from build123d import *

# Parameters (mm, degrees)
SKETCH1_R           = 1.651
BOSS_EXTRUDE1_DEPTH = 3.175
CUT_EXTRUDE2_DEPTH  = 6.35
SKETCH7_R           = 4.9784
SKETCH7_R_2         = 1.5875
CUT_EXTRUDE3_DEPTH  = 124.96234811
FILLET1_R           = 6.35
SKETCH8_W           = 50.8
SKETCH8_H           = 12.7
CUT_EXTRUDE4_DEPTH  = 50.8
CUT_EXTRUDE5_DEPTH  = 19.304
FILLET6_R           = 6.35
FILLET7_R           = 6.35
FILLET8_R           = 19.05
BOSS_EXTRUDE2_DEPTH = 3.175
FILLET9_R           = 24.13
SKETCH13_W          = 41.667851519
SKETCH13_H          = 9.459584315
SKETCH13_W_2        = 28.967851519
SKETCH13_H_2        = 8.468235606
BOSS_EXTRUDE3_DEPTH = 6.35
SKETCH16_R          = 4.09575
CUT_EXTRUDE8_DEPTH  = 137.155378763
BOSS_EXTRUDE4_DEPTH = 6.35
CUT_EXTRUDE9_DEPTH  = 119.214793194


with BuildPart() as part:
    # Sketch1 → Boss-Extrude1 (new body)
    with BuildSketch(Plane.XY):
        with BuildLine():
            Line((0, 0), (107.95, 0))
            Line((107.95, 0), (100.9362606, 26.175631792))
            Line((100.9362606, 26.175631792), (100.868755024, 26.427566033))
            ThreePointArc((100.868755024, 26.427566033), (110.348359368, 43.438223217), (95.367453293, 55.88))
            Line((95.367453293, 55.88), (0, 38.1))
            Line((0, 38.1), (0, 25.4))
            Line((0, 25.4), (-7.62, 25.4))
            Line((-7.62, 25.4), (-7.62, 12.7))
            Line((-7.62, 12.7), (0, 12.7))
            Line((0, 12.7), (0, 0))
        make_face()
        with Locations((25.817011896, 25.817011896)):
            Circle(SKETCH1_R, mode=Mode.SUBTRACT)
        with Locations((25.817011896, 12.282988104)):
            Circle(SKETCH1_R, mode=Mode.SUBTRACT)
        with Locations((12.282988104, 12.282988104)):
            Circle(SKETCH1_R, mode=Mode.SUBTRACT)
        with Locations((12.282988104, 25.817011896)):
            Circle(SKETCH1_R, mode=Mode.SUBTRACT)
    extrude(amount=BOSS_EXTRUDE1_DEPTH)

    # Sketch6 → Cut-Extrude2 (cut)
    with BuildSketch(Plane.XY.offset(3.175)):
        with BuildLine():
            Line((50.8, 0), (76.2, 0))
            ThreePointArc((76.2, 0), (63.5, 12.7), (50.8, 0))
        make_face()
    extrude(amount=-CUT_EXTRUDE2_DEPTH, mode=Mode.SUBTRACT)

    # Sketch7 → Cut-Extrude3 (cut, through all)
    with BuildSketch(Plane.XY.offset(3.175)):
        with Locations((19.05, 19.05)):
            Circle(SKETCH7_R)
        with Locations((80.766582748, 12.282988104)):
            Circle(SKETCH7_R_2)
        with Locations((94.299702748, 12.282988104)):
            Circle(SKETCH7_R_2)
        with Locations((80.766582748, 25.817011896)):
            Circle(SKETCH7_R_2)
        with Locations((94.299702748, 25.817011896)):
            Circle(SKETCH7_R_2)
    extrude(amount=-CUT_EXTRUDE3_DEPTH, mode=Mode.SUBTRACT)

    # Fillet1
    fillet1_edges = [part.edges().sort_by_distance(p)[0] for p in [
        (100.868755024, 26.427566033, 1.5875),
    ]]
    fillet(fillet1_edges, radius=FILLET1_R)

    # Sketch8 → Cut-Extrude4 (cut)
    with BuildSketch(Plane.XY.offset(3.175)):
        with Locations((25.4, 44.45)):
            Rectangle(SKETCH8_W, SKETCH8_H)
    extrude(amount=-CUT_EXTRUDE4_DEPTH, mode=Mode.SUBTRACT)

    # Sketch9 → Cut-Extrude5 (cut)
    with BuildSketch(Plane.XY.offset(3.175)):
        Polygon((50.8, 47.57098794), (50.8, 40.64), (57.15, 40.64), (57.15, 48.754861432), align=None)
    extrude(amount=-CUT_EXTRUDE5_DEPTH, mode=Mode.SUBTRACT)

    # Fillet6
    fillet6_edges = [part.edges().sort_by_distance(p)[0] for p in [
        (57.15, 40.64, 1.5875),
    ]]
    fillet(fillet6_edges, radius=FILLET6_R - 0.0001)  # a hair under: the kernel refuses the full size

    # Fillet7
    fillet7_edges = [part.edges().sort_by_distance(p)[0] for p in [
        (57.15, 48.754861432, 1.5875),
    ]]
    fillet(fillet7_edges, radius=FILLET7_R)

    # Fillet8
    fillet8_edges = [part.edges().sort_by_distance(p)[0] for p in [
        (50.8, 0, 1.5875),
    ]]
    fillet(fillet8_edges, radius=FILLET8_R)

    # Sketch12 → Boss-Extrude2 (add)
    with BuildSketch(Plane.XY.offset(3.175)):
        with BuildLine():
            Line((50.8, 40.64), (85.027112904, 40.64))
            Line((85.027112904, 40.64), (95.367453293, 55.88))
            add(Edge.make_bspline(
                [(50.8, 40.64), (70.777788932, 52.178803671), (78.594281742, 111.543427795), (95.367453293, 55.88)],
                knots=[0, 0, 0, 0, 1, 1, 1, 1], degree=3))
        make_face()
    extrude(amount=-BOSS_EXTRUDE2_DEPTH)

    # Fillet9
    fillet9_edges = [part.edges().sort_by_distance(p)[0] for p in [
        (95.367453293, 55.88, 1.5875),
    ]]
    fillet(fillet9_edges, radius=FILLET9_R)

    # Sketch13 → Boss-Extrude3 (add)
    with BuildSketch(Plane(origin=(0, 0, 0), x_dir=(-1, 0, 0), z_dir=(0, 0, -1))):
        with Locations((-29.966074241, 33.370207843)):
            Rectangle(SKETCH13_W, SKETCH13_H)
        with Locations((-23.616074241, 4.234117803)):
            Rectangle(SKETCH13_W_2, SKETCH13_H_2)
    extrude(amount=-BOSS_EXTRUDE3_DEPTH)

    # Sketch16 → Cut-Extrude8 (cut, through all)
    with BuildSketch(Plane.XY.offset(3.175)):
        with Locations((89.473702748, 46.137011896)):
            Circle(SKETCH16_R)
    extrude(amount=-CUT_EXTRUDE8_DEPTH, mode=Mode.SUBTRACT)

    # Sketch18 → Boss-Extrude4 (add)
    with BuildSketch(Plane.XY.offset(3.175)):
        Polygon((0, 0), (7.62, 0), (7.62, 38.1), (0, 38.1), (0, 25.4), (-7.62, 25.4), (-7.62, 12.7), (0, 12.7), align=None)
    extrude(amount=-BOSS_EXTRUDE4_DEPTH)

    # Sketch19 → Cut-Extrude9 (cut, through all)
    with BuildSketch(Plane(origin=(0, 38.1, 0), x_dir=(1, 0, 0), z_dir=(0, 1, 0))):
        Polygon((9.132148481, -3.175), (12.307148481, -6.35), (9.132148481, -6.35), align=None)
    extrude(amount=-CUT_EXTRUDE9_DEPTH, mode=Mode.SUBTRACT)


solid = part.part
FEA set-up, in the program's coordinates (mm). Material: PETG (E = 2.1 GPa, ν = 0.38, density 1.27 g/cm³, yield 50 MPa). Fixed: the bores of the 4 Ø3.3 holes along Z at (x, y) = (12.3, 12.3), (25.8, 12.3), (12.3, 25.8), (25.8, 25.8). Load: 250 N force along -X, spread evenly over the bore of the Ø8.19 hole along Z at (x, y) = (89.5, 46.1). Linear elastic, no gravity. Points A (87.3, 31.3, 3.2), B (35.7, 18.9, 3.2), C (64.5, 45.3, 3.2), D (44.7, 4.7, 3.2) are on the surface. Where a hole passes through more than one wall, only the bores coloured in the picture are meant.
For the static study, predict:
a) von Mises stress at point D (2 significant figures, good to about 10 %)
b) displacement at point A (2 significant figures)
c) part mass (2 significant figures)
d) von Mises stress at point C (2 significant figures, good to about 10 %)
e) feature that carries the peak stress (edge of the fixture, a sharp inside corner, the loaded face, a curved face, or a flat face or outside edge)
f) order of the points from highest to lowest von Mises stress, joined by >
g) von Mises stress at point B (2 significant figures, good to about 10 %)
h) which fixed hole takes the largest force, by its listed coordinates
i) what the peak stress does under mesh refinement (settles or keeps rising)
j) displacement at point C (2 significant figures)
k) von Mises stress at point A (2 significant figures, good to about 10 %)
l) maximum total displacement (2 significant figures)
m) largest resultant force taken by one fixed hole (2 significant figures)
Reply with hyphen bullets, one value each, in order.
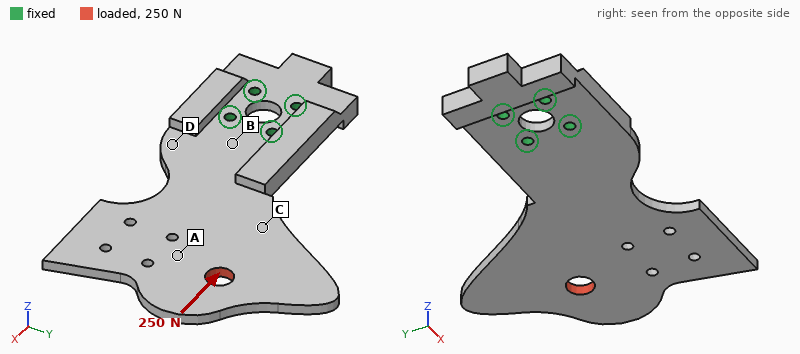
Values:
- 6.7 MPa
- 1.0 mm
- 24 g
- 4.8 MPa
- edge of the fixture
- D > C > B > A
- 2.8 MPa
- (25.8, 25.8)
- keeps rising
- 0.74 mm
- 1.3 MPa
- 1.7 mm
- 310 N
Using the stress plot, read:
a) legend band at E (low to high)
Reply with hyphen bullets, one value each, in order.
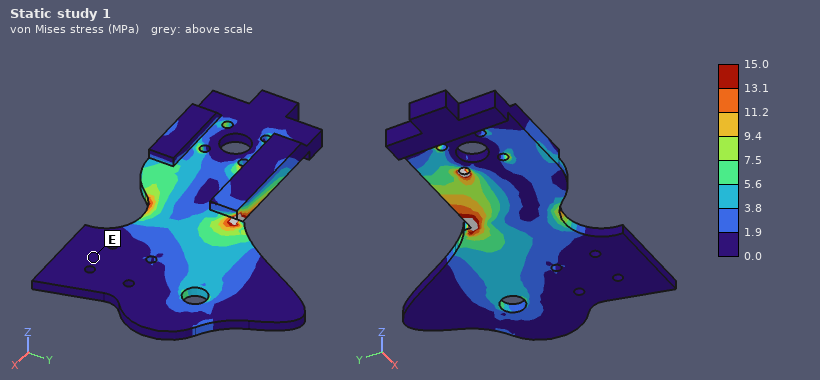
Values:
- 0.0 to 1.9 MPa
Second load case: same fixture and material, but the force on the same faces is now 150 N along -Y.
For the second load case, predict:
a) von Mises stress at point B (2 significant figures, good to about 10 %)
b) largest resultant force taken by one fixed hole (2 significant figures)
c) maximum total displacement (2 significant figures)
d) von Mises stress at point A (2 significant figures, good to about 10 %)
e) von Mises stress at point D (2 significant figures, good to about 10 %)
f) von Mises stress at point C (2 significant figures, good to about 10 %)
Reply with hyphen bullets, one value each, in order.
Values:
- 7.1 MPa
- 350 N
- 1.7 mm
- 2.1 MPa
- 9.6 MPa
- 2.4 MPa
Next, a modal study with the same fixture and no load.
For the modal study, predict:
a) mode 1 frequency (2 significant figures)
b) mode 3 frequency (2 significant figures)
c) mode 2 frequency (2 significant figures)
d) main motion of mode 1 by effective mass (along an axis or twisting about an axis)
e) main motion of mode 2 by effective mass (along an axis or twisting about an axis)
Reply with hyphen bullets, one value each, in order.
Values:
- 110 Hz
- 590 Hz
- 210 Hz
- along Z
- twisting about X
